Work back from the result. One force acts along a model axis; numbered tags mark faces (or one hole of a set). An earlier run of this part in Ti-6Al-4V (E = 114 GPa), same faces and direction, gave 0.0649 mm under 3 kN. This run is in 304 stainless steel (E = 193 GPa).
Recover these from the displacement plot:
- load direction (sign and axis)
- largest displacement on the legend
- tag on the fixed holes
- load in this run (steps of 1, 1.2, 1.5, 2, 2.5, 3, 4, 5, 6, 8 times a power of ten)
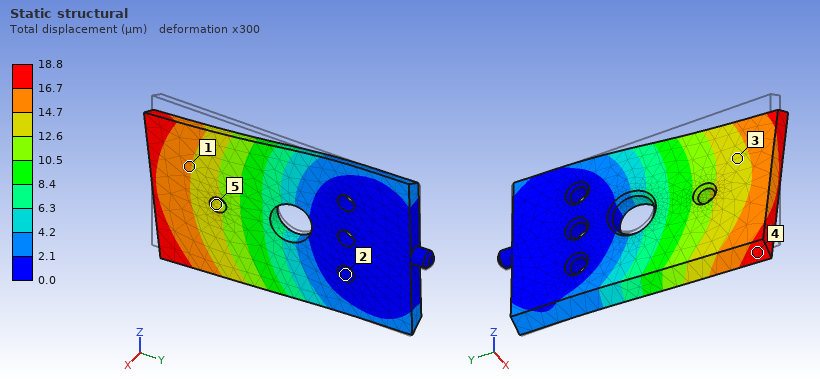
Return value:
-Z
18.8 µm
2
1.5 kN
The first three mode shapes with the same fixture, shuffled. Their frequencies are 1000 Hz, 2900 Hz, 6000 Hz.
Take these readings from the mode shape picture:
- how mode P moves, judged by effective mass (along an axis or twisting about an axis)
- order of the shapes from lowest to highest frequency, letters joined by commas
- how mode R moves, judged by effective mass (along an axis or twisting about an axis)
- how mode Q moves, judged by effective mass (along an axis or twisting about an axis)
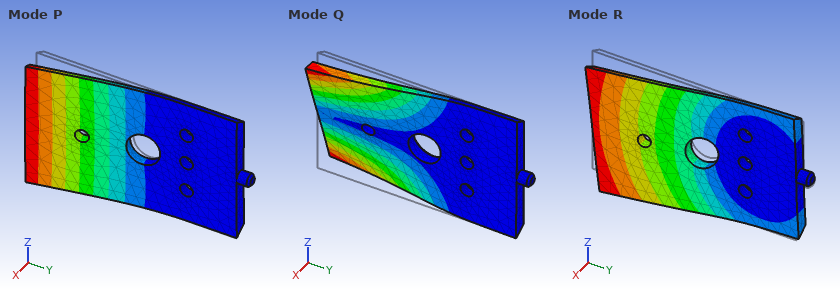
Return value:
along X
P, Q, R
along Z
twisting about Y
